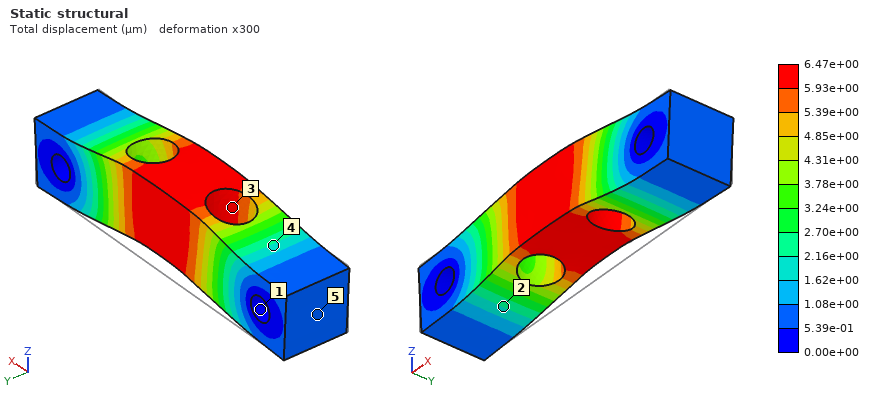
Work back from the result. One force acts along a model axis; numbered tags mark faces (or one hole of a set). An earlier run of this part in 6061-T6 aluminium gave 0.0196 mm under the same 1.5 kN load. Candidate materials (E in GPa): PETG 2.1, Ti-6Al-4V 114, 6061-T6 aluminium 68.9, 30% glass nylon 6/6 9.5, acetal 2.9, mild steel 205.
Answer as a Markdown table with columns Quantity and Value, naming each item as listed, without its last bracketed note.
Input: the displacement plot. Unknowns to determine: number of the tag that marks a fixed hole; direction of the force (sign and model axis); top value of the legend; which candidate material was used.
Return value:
| Quantity | Value |
|---|---|
| number of the tag that marks a fixed hole | 1 |
| direction of the force | +Z |
| top value of the legend | 6.47e+00 µm |
| which candidate material was used | mild steel |
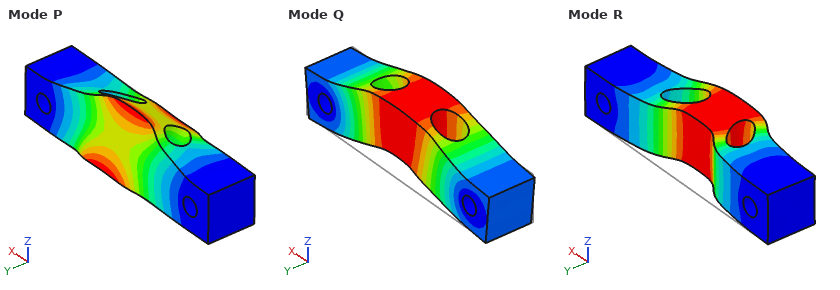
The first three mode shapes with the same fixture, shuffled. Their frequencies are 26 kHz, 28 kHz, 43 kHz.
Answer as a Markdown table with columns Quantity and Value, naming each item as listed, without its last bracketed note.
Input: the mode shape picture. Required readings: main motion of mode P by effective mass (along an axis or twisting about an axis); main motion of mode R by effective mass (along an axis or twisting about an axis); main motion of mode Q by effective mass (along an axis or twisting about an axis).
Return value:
| Quantity | Value |
|---|---|
| main motion of mode P by effective mass | twisting about X |
| main motion of mode R by effective mass | along Y |
| main motion of mode Q by effective mass | along Z |
